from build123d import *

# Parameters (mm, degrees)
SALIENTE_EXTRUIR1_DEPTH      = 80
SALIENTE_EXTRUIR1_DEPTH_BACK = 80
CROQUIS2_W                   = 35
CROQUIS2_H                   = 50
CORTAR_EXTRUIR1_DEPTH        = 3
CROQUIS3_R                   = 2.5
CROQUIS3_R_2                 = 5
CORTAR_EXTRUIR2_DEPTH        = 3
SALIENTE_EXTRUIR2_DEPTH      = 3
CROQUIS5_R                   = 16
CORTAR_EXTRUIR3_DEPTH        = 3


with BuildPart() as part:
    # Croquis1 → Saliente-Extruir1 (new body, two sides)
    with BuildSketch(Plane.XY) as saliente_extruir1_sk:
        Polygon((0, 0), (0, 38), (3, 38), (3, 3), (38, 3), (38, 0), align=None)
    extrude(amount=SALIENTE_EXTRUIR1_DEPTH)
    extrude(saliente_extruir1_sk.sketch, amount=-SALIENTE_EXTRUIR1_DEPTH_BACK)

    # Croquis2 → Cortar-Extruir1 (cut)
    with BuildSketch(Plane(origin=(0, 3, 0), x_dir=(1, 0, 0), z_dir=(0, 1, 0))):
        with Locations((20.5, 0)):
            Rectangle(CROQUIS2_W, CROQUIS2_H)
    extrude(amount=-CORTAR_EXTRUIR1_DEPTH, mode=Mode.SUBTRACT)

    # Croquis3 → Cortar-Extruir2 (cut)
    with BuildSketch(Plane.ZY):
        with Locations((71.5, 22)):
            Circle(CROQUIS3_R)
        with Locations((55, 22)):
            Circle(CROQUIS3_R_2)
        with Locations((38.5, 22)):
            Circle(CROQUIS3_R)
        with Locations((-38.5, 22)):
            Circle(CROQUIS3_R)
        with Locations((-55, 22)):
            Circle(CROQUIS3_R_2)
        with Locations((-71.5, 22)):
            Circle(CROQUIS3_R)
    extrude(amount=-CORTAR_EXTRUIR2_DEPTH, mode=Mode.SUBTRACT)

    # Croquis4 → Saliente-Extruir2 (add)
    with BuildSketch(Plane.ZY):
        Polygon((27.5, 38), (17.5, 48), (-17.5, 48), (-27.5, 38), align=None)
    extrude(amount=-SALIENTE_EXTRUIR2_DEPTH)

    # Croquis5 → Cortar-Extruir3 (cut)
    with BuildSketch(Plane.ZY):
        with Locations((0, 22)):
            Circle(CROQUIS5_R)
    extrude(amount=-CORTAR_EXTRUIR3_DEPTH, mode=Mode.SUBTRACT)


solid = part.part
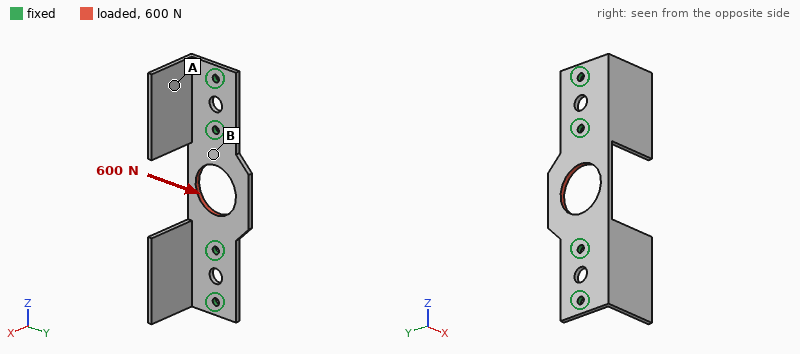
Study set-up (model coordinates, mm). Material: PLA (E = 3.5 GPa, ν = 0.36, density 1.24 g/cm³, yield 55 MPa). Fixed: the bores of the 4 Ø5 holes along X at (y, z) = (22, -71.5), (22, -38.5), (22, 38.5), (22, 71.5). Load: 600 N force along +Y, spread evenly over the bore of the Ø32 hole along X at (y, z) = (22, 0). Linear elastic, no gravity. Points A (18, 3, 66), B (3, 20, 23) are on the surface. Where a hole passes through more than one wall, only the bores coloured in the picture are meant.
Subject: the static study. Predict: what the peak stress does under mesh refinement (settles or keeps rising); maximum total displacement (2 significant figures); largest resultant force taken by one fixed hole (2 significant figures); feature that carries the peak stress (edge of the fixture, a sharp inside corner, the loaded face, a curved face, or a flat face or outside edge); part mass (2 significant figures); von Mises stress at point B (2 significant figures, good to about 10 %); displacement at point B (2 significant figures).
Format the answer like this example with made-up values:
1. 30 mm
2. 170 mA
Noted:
1. keeps rising
2. 0.14 mm
3. 360 N
4. edge of the fixture
5. 35 g
6. 5.6 MPa
7. 0.061 mm
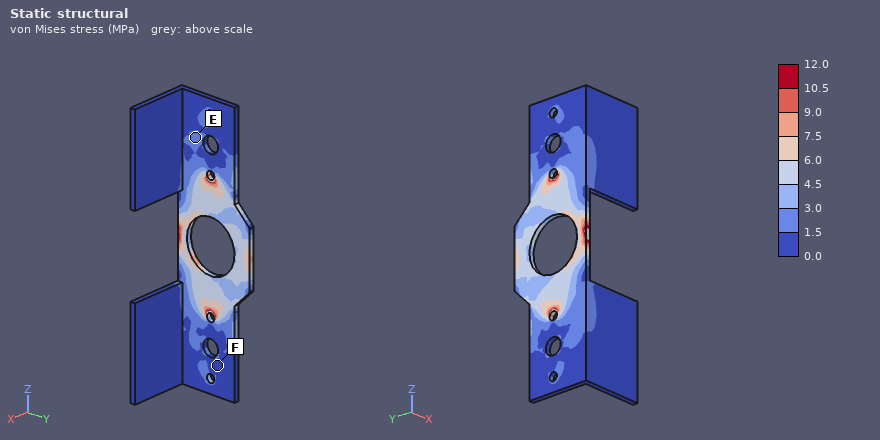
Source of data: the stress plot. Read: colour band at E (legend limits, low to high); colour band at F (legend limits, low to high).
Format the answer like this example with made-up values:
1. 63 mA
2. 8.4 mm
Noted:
1. 1.5 to 3.0 MPa
2. 0.0 to 1.5 MPa
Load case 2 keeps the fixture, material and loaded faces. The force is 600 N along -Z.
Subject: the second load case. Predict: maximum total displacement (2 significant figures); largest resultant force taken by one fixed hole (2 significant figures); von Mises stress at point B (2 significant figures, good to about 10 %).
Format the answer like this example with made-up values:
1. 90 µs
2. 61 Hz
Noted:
1. 46 µm
2. 240 N
3. 2.8 MPa
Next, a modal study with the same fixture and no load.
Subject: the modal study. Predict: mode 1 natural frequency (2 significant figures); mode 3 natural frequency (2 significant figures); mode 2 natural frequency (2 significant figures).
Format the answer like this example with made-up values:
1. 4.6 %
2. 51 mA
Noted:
1. 340 Hz
2. 630 Hz
3. 350 Hz
